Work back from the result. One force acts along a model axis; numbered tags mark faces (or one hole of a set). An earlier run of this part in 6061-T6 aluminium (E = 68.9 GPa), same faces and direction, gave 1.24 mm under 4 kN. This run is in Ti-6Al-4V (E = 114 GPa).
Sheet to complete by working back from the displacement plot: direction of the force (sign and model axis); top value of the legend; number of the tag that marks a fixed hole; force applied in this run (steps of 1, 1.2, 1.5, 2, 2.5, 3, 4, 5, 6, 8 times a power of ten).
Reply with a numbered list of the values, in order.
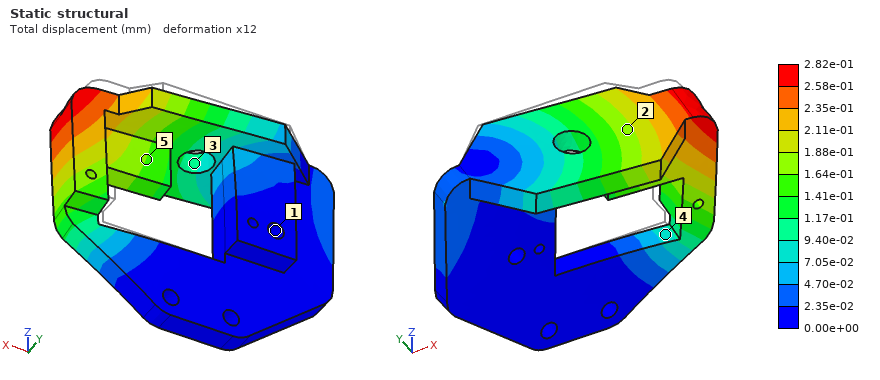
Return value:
1. -Y
2. 2.82e-01 mm
3. 1
4. 1.5 kN
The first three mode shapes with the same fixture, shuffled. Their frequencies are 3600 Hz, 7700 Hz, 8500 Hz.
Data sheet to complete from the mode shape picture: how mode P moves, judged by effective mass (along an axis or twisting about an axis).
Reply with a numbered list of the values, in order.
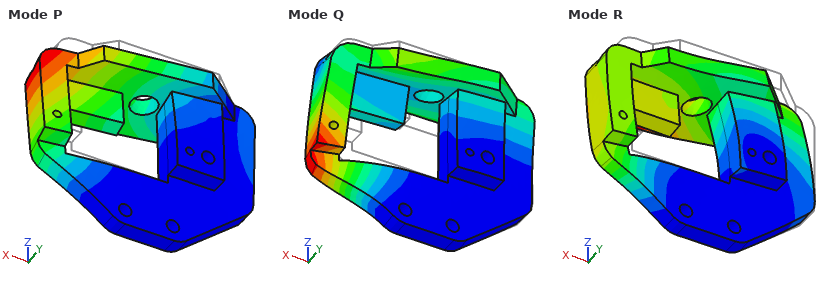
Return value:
1. along Y
